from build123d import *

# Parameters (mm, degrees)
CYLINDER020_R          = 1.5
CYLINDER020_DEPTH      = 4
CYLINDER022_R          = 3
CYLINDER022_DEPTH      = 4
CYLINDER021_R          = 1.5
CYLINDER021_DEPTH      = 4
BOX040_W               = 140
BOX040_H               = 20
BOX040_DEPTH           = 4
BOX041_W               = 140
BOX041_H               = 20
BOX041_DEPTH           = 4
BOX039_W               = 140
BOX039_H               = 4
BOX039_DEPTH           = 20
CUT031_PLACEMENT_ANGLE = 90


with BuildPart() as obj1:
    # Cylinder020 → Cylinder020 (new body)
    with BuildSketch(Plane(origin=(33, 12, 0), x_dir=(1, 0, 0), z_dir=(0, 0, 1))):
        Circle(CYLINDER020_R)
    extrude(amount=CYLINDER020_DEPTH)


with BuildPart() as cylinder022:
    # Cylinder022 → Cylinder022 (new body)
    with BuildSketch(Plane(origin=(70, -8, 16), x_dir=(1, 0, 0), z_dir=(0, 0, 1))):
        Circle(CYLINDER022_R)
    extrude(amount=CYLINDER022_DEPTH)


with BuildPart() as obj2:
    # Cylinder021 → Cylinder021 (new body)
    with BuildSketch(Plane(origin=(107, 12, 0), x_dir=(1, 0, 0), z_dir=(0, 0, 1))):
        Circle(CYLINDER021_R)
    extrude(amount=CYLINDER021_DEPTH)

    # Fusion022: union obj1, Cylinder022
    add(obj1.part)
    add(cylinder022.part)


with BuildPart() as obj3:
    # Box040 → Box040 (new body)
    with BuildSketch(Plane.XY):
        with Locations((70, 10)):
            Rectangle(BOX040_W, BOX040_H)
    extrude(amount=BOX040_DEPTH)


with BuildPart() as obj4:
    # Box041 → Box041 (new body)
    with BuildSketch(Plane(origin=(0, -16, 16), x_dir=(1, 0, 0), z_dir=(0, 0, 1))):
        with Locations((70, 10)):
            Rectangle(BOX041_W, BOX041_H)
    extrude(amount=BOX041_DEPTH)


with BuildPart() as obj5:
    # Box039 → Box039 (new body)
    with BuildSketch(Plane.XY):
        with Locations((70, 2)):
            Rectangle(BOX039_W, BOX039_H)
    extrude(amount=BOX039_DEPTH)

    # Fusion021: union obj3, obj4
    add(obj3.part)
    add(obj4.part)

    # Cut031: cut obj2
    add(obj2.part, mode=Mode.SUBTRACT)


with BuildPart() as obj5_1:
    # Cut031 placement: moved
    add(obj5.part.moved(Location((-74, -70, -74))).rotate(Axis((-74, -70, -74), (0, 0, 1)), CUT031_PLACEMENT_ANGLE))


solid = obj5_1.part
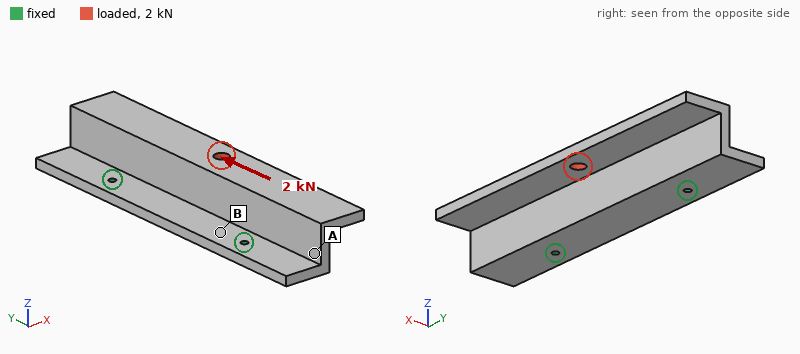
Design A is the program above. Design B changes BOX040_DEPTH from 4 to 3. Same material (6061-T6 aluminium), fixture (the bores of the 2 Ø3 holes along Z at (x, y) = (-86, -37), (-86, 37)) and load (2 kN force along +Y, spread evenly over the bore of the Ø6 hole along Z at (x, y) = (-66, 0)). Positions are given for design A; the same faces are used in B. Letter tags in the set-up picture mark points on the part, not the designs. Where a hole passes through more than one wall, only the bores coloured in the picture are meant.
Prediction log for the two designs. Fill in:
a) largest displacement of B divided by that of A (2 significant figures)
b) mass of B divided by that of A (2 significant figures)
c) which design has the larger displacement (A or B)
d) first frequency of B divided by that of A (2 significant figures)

1.4
0.92
B
0.70
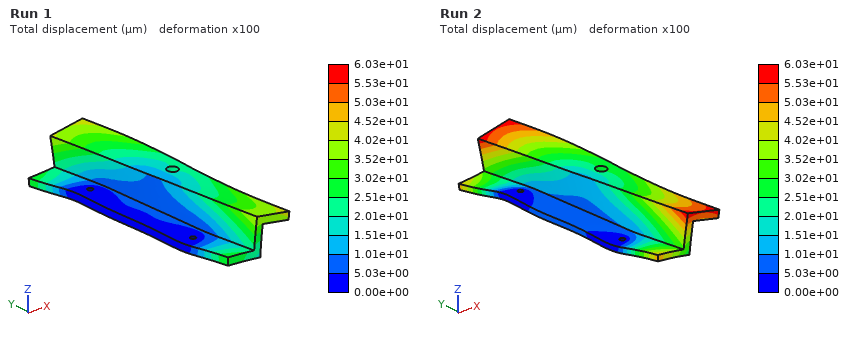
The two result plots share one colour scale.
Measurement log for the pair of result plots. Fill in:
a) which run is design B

Run 2
